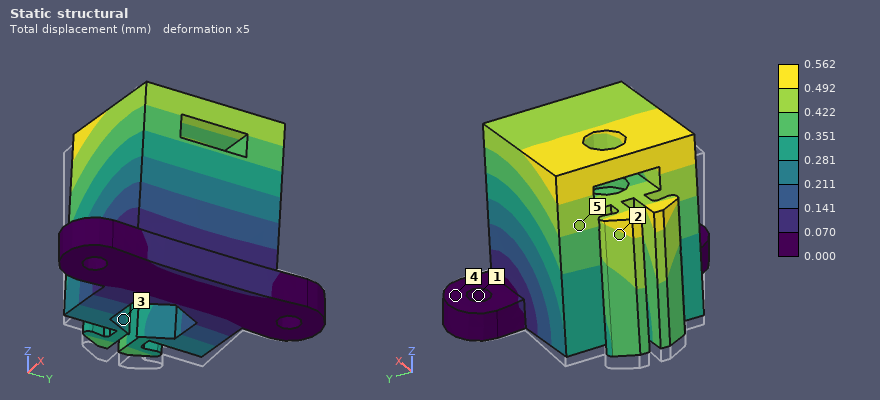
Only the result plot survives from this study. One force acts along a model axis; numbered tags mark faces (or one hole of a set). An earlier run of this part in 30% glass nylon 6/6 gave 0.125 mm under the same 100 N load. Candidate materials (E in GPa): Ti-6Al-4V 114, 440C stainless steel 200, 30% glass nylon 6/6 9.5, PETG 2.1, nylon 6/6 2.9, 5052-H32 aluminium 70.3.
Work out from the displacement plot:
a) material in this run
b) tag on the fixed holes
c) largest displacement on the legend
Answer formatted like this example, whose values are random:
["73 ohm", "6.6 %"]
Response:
["PETG", "1", "0.562 mm"]
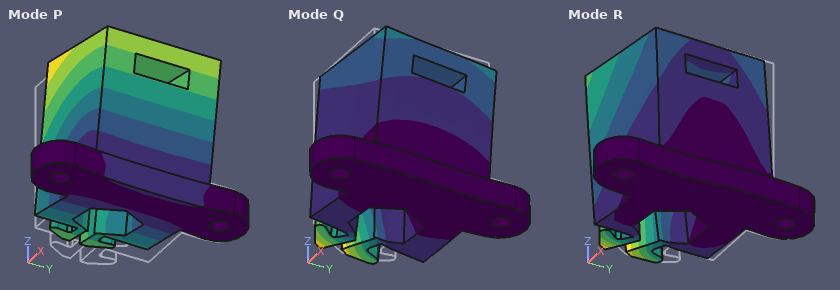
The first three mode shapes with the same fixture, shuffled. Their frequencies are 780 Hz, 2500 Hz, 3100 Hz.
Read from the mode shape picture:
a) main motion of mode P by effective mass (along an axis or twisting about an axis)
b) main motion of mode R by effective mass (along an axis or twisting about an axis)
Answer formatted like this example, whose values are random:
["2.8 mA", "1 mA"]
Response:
["along X", "along Y"]
